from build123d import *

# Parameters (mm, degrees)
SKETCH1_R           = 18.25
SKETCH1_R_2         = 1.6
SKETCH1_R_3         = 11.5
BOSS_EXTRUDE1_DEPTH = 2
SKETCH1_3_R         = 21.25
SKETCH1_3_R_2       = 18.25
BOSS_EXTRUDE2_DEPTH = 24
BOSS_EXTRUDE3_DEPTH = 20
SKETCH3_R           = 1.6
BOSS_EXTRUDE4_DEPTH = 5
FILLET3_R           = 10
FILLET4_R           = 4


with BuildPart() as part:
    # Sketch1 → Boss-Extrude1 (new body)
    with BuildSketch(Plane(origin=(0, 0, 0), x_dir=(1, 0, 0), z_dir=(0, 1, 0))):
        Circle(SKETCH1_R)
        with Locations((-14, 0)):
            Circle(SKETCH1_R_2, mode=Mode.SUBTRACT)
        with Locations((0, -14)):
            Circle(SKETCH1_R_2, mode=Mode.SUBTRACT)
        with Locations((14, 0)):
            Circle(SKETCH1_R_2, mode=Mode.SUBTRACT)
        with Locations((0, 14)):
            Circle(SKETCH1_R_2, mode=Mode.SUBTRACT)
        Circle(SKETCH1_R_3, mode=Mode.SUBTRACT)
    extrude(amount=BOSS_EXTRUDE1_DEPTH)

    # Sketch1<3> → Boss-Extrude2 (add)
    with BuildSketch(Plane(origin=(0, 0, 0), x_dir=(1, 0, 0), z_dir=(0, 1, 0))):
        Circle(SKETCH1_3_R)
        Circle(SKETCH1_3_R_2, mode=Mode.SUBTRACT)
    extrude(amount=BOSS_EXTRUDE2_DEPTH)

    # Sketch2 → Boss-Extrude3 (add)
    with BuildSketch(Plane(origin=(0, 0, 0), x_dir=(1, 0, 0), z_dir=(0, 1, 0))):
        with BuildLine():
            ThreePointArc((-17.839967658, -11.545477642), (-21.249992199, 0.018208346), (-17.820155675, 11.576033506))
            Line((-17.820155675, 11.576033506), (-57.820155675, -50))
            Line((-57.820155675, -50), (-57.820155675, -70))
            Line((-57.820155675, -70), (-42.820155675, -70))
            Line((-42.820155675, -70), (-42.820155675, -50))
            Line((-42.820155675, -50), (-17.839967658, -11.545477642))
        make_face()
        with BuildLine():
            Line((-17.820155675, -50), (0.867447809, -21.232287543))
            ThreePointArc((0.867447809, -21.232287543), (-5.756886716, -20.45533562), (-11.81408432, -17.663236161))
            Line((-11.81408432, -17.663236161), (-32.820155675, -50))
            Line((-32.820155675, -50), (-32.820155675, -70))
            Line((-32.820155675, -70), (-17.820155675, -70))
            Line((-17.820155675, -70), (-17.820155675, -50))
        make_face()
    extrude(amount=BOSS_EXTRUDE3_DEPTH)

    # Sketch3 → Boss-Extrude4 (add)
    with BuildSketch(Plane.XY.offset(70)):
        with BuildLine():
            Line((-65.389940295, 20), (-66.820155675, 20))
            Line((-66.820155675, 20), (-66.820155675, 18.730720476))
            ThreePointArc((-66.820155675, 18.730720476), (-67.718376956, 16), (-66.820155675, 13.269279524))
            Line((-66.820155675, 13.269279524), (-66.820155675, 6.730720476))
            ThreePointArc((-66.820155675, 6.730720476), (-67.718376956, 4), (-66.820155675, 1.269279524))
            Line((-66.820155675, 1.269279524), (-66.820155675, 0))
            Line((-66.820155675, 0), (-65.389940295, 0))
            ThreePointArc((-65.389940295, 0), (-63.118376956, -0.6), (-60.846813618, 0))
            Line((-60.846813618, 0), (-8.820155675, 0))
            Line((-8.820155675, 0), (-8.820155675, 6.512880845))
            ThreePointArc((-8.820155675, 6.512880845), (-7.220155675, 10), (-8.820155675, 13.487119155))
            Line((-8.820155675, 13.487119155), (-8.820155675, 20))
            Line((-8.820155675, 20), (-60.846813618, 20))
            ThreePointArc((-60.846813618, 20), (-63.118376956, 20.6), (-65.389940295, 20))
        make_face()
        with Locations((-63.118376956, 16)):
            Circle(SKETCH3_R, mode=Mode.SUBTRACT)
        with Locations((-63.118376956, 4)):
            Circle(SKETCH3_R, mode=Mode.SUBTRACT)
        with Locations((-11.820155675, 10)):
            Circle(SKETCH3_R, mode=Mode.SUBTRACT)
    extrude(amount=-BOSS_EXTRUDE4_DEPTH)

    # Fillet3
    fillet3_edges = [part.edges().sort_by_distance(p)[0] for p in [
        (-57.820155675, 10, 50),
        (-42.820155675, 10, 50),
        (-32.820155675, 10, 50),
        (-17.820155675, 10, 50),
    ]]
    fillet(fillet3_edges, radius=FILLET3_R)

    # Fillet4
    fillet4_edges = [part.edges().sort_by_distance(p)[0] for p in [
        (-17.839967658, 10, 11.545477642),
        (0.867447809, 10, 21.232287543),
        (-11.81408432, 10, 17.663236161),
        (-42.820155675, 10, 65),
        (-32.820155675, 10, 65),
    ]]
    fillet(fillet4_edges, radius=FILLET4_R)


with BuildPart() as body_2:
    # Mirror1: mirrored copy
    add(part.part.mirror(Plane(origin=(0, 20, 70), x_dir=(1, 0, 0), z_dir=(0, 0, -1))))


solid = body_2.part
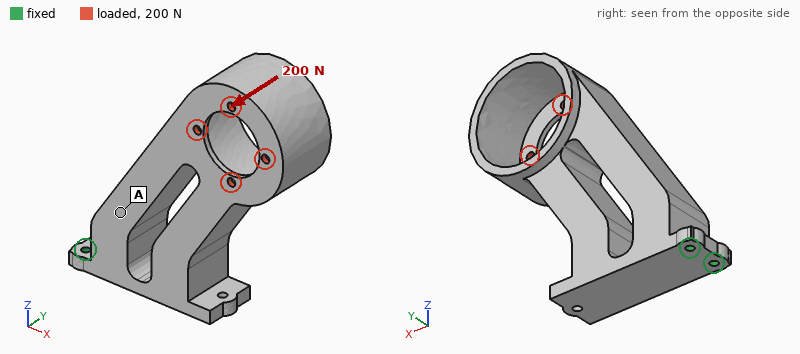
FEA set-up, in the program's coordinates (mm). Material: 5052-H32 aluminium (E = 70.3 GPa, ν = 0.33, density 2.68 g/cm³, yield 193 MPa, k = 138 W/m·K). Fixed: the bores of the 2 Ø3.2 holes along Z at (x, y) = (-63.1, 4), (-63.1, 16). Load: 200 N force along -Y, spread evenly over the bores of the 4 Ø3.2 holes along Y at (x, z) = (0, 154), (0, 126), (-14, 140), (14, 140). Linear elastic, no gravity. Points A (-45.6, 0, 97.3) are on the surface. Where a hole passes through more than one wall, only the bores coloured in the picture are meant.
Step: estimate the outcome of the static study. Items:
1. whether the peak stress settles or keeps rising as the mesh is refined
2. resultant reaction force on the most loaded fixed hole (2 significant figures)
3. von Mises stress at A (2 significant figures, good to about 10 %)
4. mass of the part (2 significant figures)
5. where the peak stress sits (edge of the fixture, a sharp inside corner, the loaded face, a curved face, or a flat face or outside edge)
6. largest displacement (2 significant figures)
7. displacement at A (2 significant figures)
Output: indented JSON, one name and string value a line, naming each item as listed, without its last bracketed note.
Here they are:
{
  "whether the peak stress settles or keeps rising as the mesh is refined": "keeps rising",
  "resultant reaction force on the most loaded fixed hole": "1.3 kN",
  "von Mises stress at A": "12 MPa",
  "mass of the part": "130 g",
  "where the peak stress sits": "edge of the fixture",
  "largest displacement": "0.24 mm",
  "displacement at A": "0.053 mm"
}
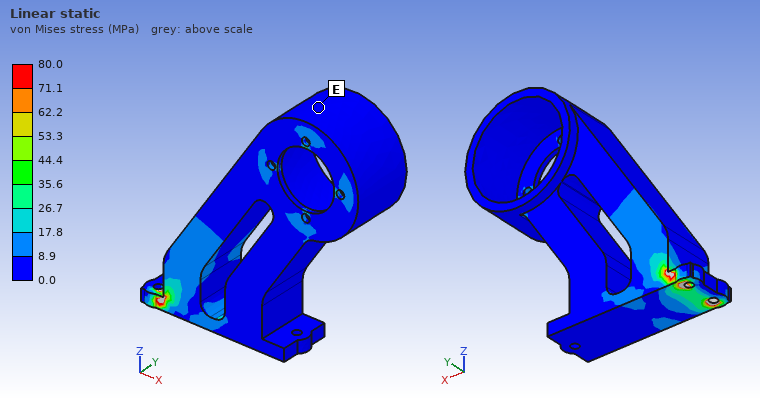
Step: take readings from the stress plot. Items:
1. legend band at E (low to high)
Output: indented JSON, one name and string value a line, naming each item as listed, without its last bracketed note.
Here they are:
{
  "legend band at E": "0.0 to 8.9 MPa"
}
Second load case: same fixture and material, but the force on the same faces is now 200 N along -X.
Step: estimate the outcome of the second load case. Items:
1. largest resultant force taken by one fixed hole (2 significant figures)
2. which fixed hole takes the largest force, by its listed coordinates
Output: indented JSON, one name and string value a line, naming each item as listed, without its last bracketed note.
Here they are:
{
  "largest resultant force taken by one fixed hole": "240 N",
  "which fixed hole takes the largest force, by its listed coordinates": "(-63.1, 4)"
}
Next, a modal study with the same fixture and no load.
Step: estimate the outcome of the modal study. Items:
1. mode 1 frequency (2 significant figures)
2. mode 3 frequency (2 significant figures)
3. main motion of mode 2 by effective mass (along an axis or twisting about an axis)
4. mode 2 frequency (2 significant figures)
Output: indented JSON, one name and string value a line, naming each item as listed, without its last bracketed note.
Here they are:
{
  "mode 1 frequency": "330 Hz",
  "mode 3 frequency": "2600 Hz",
  "main motion of mode 2 by effective mass": "along Y",
  "mode 2 frequency": "760 Hz"
}
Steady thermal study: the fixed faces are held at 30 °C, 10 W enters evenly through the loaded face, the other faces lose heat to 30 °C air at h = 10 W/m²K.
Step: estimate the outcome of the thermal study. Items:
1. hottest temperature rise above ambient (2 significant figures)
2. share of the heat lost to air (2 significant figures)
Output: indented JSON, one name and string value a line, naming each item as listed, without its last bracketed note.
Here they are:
{
  "hottest temperature rise above ambient": "25 K",
  "share of the heat lost to air": "23 %"
}
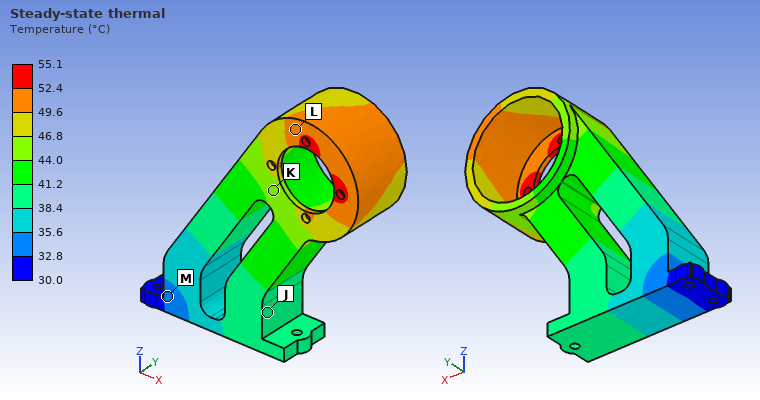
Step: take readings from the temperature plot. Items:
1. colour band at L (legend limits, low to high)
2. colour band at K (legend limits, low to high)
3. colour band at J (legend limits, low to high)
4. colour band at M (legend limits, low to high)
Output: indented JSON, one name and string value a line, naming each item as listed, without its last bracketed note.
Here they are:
{
  "colour band at L": "49.6 to 52.4 °C",
  "colour band at K": "44.0 to 46.8 °C",
  "colour band at J": "38.4 to 41.2 °C",
  "colour band at M": "32.8 to 35.6 °C"
}
